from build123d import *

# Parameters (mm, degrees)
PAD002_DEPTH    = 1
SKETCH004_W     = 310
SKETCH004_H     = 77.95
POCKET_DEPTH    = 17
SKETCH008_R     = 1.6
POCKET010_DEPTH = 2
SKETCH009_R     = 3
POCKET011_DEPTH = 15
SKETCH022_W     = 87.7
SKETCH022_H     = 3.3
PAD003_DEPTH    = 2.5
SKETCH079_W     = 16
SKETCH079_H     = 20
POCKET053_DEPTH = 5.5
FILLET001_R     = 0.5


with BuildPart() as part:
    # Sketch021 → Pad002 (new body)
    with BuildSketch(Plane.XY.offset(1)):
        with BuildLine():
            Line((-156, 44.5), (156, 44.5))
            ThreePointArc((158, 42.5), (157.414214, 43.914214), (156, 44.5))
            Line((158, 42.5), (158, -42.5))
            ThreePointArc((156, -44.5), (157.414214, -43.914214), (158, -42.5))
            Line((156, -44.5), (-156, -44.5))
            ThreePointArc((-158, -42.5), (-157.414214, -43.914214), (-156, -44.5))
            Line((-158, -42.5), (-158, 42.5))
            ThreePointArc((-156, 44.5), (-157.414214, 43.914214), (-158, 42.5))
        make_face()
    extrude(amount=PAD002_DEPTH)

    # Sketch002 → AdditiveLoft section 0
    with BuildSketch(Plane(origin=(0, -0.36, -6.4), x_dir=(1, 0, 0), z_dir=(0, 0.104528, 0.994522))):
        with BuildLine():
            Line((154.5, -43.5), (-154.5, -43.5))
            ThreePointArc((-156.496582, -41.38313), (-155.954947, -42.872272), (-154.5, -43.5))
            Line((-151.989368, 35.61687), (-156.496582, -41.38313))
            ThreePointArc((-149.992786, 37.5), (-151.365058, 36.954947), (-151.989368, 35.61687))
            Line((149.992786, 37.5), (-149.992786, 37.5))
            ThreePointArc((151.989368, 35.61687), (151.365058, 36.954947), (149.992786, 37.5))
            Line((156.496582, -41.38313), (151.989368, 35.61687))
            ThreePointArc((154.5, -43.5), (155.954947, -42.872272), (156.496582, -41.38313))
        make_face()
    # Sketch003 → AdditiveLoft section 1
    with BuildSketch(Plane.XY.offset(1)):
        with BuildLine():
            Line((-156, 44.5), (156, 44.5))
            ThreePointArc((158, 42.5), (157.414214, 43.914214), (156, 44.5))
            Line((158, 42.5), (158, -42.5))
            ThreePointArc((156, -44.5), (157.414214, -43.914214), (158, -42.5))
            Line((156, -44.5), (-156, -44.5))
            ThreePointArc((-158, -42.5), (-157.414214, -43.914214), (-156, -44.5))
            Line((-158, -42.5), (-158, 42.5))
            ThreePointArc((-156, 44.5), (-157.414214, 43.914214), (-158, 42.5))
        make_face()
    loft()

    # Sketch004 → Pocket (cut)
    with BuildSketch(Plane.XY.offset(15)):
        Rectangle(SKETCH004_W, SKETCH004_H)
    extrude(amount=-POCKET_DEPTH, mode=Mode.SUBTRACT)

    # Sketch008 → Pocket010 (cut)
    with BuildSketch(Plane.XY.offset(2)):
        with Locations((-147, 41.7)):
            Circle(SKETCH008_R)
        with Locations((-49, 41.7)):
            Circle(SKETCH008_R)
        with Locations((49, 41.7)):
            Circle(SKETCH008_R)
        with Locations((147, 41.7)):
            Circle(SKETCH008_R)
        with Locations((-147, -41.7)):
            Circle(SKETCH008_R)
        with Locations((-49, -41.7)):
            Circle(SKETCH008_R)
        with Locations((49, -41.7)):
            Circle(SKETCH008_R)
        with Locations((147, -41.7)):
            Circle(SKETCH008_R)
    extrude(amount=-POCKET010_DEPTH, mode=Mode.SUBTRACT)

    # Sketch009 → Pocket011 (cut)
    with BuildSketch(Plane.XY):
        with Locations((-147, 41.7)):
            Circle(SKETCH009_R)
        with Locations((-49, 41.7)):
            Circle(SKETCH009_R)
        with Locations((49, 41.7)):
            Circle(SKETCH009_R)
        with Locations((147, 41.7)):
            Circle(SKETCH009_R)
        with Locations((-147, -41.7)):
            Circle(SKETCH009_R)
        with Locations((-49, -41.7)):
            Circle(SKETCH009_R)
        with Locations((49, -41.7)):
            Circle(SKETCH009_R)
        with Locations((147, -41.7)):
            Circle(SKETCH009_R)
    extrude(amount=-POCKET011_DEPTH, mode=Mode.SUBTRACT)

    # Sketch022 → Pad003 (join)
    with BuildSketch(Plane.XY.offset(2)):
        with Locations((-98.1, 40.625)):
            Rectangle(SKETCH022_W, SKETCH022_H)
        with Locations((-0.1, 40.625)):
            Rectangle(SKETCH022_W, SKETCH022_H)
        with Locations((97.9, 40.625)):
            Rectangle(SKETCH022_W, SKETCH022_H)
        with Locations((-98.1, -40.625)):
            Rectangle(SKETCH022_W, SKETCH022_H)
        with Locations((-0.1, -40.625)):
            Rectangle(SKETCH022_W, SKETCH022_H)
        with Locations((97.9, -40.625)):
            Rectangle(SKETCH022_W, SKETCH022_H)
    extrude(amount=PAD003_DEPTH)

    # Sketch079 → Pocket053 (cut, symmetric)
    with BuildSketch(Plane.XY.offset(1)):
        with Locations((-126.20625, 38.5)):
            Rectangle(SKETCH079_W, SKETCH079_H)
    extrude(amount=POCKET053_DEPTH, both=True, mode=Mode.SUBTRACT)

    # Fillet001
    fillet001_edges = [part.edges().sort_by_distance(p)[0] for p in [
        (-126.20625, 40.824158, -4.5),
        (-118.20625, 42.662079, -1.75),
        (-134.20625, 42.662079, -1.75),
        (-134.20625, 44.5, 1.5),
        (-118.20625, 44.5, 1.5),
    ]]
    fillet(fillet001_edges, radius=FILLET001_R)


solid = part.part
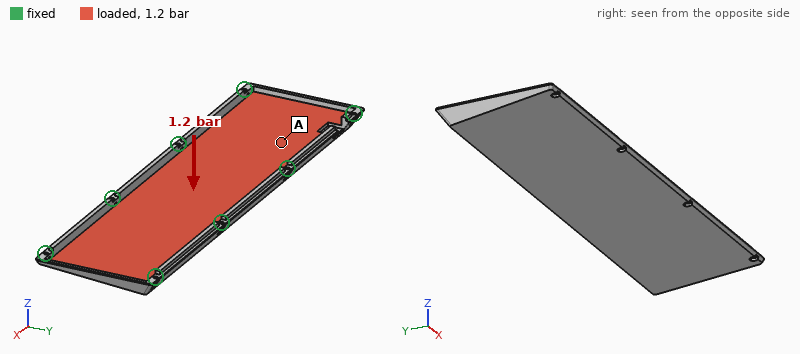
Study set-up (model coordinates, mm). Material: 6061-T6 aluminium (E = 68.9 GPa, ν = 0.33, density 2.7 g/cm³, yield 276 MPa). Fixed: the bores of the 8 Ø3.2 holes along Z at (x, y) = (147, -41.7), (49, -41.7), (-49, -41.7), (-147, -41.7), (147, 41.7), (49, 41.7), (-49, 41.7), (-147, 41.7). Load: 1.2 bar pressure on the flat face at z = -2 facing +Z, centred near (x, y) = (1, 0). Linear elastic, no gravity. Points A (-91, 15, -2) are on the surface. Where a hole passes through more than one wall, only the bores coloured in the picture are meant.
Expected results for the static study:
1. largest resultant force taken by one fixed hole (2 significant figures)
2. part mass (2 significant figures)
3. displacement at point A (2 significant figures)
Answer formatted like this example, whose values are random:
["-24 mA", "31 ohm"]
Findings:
["1.0 kN", "340 g", "0.12 mm"]
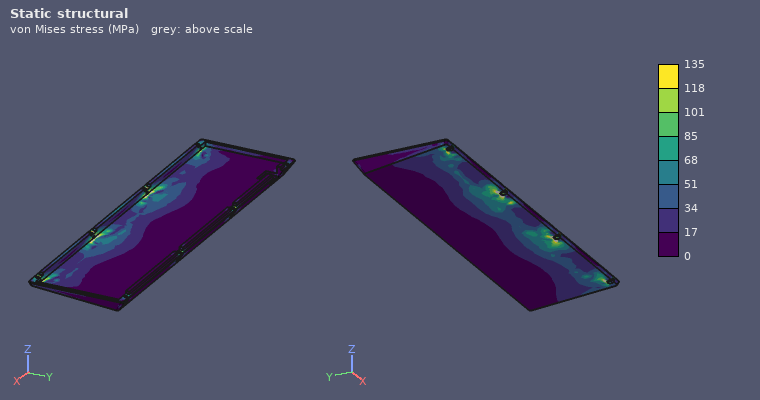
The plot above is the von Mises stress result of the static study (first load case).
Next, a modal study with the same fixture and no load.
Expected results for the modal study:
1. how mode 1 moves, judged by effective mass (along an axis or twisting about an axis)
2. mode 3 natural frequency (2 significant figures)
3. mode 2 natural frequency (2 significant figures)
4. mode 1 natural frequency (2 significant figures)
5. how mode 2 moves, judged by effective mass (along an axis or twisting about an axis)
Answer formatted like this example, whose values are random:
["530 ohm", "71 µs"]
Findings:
["along Z", "1800 Hz", "1600 Hz", "1400 Hz", "twisting about Y"]
